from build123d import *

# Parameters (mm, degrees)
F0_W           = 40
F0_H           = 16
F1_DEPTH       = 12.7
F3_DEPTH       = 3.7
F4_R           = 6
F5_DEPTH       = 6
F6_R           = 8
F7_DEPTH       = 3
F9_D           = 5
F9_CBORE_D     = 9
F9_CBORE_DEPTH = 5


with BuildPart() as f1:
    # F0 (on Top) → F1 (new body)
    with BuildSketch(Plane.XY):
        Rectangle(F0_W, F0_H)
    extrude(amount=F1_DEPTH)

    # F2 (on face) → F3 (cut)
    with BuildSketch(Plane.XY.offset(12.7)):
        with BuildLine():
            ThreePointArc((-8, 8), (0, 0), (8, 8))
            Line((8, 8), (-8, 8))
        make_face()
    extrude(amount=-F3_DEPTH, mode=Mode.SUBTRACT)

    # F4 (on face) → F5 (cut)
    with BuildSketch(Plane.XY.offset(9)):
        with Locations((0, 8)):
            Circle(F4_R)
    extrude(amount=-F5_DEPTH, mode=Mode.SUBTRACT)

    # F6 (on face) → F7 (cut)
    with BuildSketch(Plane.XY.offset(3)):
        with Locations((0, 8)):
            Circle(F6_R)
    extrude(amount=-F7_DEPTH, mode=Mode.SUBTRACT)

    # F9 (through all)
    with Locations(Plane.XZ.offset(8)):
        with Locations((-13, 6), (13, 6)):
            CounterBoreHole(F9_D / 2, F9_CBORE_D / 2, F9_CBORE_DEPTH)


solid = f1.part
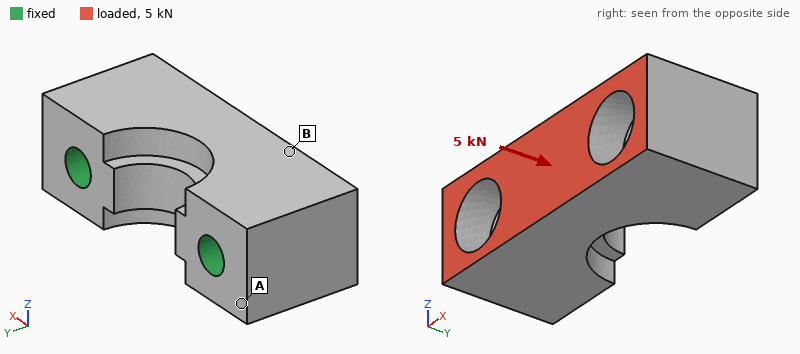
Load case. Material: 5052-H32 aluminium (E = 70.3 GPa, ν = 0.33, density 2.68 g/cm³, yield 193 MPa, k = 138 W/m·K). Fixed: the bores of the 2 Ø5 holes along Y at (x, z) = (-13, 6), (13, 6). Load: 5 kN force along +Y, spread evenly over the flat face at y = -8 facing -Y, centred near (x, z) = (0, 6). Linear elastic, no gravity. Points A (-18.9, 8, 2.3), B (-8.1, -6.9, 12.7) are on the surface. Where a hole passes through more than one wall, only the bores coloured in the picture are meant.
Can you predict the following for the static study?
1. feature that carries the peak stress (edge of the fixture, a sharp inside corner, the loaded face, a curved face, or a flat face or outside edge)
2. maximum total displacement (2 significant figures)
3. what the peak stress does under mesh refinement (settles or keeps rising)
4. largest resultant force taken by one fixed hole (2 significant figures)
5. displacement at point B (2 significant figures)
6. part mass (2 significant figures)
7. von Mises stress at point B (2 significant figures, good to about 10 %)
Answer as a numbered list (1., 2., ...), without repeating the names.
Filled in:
1. edge of the fixture
2. 6.0 µm
3. keeps rising
4. 2.6 kN
5. 4.0 µm
6. 16 g
7. 13 MPa
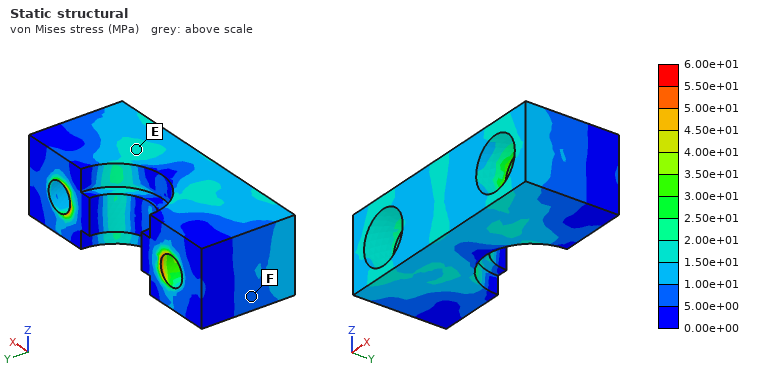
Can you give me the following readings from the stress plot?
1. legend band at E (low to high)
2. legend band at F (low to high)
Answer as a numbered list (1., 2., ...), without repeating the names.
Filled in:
1. 1.50e+01 to 2.00e+01 MPa
2. 5.00e+00 to 1.00e+01 MPa
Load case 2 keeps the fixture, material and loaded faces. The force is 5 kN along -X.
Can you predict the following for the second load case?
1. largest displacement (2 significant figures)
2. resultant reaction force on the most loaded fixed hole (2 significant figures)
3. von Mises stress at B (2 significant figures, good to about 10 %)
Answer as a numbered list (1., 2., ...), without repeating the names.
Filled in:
1. 14 µm
2. 2.8 kN
3. 29 MPa
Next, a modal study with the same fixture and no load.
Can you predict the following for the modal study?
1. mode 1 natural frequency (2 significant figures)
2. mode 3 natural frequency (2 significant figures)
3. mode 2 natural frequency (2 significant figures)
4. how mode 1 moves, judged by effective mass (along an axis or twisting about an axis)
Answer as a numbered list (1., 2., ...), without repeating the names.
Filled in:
1. 36 kHz
2. 56 kHz
3. 54 kHz
4. along Z
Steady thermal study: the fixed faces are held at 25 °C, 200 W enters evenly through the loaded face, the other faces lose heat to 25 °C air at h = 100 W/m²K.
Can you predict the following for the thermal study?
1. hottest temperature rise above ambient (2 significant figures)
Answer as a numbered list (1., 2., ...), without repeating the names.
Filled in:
1. 51 K
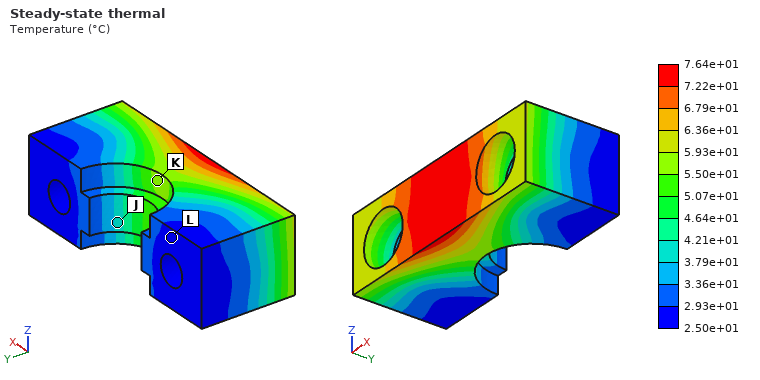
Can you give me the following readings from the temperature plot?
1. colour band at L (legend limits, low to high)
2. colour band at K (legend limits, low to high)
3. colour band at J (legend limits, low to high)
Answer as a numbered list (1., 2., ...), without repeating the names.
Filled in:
1. 2.50e+01 to 2.93e+01 °C
2. 5.50e+01 to 5.93e+01 °C
3. 3.79e+01 to 4.21e+01 °C
